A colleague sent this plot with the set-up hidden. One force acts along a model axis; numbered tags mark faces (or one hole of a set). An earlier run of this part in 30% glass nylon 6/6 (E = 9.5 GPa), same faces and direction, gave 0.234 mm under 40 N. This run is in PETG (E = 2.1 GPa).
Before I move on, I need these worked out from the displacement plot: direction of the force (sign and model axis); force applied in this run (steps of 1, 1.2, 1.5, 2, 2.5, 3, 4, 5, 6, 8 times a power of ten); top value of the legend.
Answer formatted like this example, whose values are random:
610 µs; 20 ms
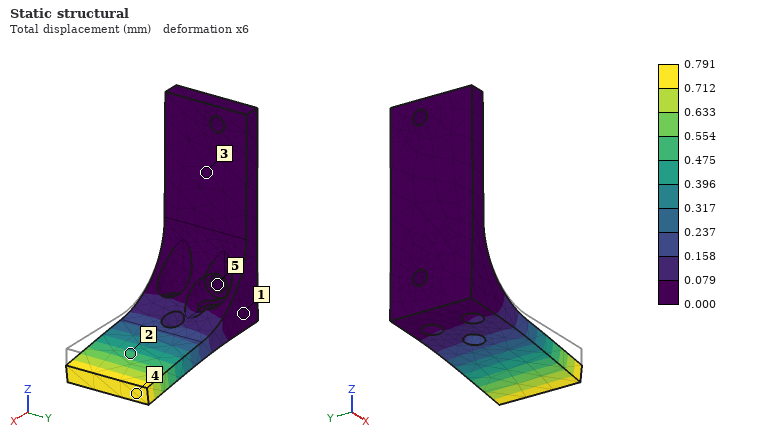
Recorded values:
-Z; 30 N; 0.791 mm
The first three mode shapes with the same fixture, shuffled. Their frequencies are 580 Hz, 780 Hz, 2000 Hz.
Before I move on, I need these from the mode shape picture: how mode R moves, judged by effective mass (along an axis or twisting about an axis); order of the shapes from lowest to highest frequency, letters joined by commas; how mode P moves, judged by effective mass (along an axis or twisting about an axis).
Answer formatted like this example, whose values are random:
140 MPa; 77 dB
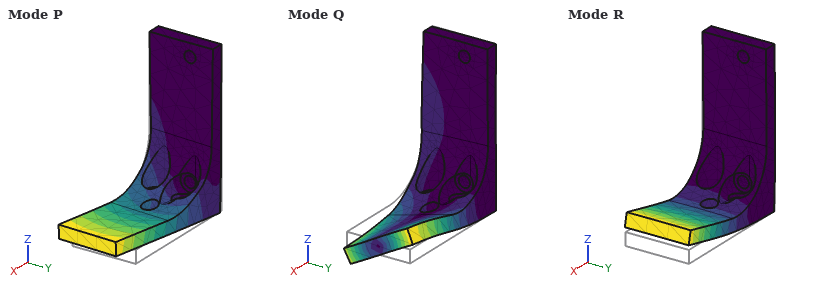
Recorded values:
along Z; R, P, Q; along Y
